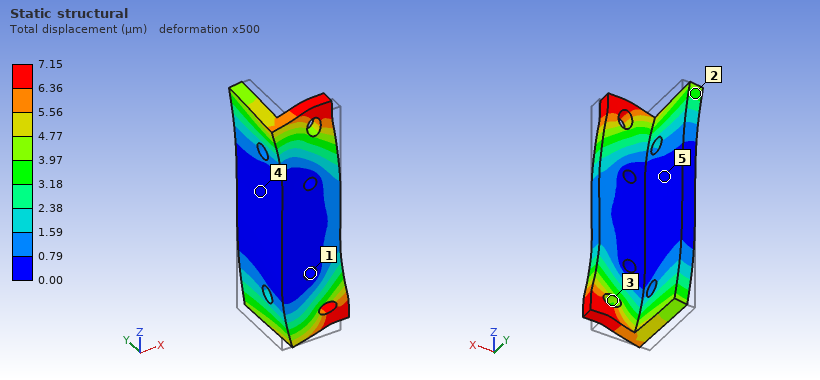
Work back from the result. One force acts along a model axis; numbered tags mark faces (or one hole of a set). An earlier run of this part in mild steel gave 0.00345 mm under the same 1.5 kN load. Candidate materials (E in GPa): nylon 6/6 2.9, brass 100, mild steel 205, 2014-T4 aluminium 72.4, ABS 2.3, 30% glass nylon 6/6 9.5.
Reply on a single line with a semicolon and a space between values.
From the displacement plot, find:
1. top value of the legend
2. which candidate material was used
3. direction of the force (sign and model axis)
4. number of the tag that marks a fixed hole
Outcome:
7.15 µm; brass; +Z; 1
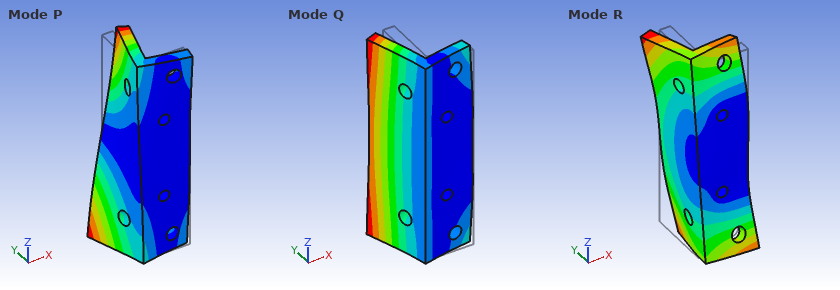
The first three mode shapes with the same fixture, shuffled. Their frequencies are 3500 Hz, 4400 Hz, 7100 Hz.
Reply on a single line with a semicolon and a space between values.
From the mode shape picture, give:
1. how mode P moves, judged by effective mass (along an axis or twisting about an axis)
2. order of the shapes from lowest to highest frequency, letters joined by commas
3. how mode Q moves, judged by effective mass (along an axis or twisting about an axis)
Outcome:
twisting about Y; Q, P, R; along X
